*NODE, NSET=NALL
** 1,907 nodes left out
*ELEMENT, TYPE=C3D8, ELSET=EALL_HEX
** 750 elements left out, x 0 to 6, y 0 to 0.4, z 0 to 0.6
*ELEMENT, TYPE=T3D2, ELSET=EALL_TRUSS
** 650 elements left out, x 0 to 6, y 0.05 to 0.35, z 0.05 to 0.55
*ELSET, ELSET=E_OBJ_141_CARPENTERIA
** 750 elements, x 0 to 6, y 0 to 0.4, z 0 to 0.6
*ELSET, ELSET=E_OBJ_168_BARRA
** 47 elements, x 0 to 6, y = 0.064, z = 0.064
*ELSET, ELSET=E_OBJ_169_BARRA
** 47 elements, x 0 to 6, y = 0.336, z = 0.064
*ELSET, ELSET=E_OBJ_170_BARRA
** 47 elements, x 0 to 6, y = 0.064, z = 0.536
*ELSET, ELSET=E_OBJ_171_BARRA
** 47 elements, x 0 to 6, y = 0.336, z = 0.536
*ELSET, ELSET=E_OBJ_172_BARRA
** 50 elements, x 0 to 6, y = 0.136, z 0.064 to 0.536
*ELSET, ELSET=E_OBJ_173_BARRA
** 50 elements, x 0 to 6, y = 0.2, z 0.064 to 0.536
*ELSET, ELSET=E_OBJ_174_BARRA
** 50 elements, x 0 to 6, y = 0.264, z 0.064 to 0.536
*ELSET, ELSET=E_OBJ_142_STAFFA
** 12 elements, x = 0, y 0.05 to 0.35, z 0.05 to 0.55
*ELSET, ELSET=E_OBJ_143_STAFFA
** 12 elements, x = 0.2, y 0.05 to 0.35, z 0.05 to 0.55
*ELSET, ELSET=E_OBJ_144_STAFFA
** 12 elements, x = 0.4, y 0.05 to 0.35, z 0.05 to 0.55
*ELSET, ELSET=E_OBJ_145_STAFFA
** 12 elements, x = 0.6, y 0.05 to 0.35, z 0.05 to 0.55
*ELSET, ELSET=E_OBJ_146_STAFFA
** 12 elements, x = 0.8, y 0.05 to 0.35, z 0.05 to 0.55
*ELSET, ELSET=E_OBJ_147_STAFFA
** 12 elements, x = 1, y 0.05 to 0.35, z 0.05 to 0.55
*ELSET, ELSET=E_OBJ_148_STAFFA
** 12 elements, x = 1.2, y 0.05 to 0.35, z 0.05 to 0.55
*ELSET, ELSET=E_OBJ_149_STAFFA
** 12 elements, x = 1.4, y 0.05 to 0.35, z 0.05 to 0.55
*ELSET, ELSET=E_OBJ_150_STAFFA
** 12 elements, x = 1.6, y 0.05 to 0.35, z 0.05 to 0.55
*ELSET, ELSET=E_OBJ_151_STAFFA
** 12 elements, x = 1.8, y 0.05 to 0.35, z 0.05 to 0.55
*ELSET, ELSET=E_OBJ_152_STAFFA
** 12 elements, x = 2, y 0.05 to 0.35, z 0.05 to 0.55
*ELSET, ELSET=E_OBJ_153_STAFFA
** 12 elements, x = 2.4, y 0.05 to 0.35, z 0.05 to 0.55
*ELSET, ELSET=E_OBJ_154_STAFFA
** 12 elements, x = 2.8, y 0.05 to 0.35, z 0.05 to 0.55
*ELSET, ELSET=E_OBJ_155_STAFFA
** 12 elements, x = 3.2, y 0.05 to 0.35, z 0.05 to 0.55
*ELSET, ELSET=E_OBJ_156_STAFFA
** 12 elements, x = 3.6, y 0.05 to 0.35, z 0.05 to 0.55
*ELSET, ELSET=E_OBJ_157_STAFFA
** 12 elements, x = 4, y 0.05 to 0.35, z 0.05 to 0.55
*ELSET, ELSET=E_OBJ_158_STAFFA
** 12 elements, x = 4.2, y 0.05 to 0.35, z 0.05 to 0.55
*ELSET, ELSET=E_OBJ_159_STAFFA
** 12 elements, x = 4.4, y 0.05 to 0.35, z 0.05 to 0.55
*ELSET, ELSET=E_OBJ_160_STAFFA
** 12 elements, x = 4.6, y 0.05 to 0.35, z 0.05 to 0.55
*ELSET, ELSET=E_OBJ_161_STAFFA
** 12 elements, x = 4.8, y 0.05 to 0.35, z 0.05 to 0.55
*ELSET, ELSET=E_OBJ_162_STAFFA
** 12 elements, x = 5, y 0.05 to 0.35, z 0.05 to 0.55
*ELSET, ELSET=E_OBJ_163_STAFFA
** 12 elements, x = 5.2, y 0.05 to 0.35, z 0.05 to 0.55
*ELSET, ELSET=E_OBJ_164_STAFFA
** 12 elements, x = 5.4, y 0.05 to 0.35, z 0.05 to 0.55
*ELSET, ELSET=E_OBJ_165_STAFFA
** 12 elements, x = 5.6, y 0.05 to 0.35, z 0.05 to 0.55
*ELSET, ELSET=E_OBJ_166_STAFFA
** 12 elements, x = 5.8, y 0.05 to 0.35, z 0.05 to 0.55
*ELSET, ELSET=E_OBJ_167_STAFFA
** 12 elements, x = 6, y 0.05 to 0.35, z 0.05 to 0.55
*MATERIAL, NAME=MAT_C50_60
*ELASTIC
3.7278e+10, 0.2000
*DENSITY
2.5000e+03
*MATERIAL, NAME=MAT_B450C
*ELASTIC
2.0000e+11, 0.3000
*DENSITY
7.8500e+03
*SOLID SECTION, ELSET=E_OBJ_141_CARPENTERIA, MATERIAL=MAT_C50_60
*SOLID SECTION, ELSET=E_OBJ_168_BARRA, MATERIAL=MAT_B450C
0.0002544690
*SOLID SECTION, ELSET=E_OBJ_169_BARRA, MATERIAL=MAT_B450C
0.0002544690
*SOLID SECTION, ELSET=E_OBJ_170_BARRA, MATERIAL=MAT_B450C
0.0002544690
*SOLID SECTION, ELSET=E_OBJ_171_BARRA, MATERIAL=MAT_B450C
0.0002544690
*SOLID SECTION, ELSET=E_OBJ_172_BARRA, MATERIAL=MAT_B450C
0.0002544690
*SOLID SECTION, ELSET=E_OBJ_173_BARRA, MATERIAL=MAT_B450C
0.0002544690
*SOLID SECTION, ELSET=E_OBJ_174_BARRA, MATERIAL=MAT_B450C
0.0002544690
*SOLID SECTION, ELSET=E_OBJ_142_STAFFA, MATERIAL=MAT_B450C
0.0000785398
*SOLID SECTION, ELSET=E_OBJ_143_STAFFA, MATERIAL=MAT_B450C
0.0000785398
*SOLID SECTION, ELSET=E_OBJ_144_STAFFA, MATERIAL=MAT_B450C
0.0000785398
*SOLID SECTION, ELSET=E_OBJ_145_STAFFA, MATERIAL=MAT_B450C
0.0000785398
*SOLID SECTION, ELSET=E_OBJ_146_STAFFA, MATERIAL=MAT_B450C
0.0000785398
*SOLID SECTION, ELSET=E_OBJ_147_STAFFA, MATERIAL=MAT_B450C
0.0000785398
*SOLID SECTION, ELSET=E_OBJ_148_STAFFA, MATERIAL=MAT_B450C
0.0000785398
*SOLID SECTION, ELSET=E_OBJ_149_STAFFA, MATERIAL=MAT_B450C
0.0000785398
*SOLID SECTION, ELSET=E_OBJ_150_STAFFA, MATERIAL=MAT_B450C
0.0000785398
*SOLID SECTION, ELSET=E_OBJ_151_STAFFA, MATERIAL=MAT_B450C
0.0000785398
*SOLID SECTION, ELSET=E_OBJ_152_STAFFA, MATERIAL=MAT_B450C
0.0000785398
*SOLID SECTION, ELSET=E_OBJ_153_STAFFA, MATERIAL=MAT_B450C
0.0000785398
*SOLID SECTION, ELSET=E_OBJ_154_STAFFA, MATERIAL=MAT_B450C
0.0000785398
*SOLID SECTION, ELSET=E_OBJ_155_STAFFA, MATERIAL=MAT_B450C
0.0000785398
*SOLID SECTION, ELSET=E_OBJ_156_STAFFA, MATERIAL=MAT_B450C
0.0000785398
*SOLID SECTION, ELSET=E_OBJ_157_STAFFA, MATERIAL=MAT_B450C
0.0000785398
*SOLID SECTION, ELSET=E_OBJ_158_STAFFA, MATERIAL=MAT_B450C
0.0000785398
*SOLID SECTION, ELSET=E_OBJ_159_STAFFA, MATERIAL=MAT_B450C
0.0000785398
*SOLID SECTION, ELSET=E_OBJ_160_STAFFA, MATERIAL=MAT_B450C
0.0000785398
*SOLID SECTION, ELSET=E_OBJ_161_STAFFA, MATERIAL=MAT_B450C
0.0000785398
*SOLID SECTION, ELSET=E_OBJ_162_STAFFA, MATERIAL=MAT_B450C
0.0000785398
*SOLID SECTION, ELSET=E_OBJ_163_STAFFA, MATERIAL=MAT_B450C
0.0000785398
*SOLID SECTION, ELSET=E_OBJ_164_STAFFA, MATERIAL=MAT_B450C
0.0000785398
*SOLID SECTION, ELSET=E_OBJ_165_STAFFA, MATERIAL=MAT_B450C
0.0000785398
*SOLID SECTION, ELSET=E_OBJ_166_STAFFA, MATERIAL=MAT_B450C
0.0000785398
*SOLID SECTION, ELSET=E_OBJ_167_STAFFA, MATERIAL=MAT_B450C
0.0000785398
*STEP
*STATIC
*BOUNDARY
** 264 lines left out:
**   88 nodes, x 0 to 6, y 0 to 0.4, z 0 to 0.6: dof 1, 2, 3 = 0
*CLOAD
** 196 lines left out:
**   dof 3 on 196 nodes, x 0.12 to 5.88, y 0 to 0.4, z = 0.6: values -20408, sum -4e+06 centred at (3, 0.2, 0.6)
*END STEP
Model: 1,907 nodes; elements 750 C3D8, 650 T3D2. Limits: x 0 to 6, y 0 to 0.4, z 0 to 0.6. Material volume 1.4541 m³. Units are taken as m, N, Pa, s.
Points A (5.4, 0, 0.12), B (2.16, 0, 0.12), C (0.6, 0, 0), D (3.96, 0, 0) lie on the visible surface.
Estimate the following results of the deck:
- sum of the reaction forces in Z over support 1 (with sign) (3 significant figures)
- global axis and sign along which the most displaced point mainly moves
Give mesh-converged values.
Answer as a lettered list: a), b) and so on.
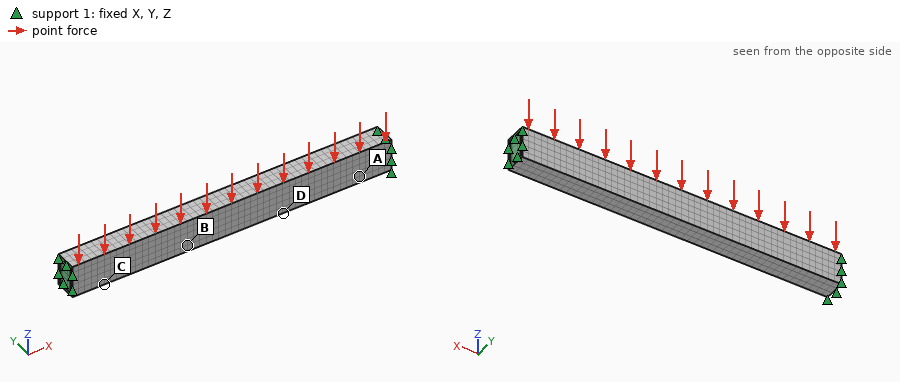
a) 4.00e+06 N
b) -Z
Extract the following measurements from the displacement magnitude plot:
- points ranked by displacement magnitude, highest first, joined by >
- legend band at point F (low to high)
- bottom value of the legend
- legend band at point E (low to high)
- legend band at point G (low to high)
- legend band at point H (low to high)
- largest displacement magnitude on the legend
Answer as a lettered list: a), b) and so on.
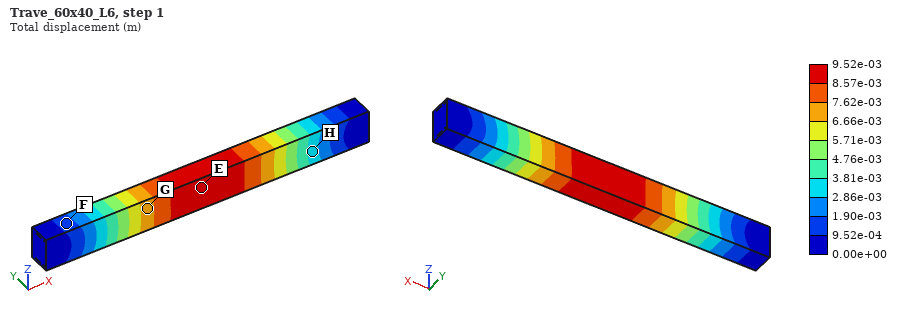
a) E > G > H > F
b) 9.52e-04 to 1.90e-03 m
c) 0.00e+00 m
d) 8.57e-03 to 9.52e-03 m
e) 6.66e-03 to 7.62e-03 m
f) 2.86e-03 to 3.81e-03 m
g) 9.52e-03 m
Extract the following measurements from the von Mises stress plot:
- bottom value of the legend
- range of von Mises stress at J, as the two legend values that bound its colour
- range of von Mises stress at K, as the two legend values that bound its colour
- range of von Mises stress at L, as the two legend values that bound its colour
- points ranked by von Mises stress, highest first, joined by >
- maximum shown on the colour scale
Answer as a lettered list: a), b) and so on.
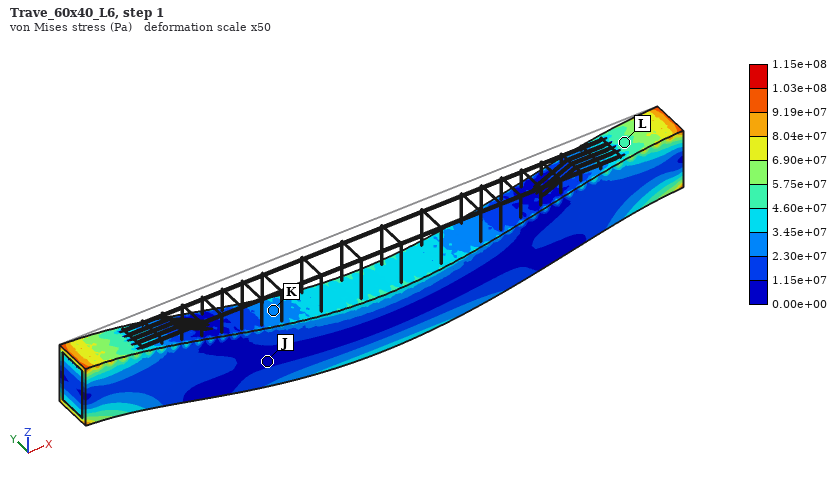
a) 0.00e+00 Pa
b) 0.00e+00 to 1.15e+07 Pa
c) 2.30e+07 to 3.45e+07 Pa
d) 4.60e+07 to 5.75e+07 Pa
e) L > K > J
f) 1.15e+08 Pa
